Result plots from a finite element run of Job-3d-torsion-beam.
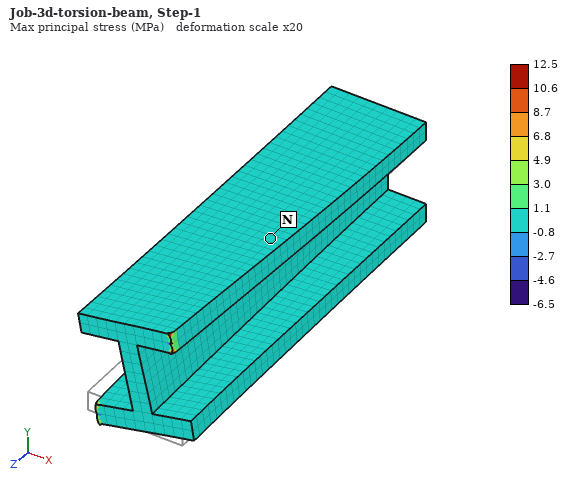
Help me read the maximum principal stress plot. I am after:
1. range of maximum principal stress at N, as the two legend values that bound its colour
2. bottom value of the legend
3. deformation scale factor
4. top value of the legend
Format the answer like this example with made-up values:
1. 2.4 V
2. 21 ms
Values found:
1. -0.8 to 1.1 MPa
2. -6.5 MPa
3. 20
4. 12.5 MPa
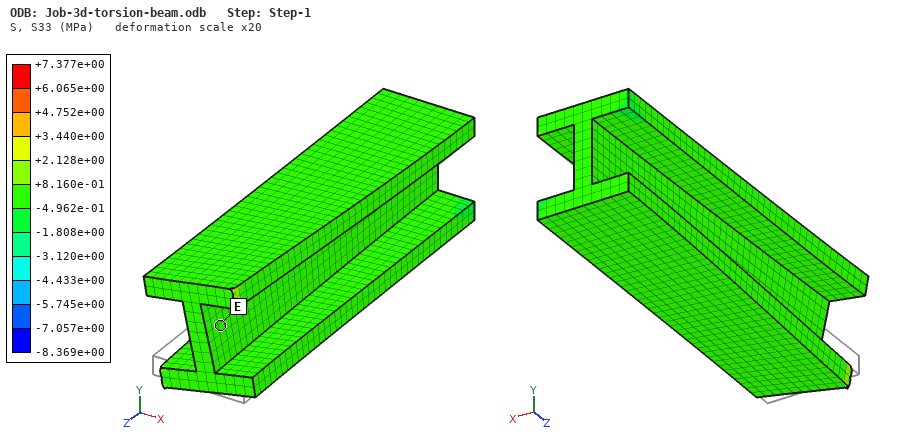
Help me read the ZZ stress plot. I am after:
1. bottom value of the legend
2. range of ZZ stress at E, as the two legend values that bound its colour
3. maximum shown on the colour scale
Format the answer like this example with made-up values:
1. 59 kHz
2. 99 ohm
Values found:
1. -8.369e+00 MPa
2. -4.962e-01 to +8.160e-01 MPa
3. +7.377e+00 MPa
